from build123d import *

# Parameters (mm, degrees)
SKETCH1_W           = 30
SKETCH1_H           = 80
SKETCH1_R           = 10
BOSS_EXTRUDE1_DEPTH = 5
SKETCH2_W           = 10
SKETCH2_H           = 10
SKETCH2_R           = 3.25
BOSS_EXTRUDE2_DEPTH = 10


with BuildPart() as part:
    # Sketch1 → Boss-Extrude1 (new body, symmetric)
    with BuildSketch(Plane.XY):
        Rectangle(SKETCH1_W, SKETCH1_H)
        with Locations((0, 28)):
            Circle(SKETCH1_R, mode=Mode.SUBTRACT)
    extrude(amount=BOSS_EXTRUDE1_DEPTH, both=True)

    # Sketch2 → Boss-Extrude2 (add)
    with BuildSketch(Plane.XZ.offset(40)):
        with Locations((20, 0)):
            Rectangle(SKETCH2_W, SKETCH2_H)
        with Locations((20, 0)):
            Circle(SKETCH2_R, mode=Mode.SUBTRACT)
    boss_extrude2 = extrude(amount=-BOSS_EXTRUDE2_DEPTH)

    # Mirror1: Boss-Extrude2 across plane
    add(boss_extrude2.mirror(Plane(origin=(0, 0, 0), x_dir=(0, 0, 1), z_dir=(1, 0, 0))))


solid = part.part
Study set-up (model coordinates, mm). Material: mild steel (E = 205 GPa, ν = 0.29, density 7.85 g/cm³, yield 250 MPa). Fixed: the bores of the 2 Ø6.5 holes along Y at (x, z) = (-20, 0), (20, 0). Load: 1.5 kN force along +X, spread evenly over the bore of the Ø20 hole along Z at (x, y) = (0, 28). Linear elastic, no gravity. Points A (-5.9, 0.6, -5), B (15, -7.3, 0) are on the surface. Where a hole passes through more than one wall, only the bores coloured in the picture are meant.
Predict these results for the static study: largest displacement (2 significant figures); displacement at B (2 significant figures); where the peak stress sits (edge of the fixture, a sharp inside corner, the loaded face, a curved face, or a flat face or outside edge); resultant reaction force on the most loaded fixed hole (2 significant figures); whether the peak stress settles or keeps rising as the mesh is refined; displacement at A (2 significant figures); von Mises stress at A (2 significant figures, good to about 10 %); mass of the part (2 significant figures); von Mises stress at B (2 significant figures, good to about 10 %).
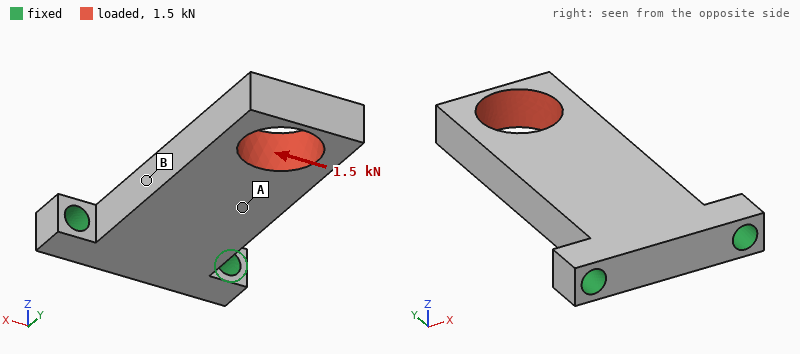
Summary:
59 µm
13 µm
edge of the fixture
3.0 kN
keeps rising
16 µm
15 MPa
170 g
35 MPa
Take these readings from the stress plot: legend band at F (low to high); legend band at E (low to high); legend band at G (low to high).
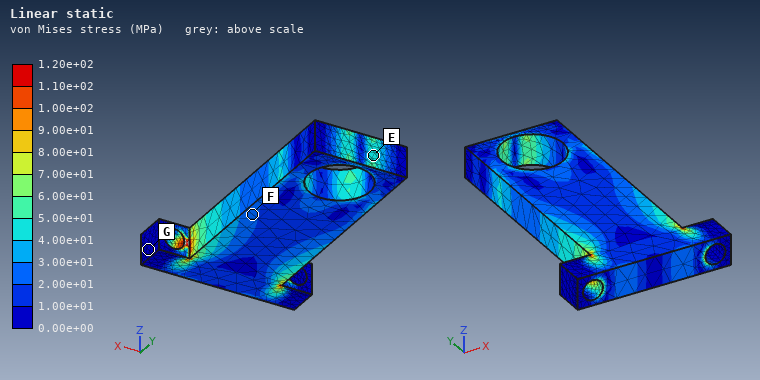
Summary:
2.00e+01 to 3.00e+01 MPa
4.00e+01 to 5.00e+01 MPa
0.00e+00 to 1.00e+01 MPa
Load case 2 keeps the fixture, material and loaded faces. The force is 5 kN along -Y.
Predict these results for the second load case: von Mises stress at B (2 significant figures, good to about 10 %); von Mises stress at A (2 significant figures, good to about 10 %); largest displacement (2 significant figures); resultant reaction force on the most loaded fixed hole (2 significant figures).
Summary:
17 MPa
15 MPa
20 µm
2.6 kN
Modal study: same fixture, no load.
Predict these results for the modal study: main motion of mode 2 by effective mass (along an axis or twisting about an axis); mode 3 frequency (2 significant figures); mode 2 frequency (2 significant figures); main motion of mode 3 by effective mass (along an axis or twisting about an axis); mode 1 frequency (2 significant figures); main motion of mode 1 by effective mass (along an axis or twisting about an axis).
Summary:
along X
6300 Hz
4300 Hz
twisting about Y
1400 Hz
along Z
